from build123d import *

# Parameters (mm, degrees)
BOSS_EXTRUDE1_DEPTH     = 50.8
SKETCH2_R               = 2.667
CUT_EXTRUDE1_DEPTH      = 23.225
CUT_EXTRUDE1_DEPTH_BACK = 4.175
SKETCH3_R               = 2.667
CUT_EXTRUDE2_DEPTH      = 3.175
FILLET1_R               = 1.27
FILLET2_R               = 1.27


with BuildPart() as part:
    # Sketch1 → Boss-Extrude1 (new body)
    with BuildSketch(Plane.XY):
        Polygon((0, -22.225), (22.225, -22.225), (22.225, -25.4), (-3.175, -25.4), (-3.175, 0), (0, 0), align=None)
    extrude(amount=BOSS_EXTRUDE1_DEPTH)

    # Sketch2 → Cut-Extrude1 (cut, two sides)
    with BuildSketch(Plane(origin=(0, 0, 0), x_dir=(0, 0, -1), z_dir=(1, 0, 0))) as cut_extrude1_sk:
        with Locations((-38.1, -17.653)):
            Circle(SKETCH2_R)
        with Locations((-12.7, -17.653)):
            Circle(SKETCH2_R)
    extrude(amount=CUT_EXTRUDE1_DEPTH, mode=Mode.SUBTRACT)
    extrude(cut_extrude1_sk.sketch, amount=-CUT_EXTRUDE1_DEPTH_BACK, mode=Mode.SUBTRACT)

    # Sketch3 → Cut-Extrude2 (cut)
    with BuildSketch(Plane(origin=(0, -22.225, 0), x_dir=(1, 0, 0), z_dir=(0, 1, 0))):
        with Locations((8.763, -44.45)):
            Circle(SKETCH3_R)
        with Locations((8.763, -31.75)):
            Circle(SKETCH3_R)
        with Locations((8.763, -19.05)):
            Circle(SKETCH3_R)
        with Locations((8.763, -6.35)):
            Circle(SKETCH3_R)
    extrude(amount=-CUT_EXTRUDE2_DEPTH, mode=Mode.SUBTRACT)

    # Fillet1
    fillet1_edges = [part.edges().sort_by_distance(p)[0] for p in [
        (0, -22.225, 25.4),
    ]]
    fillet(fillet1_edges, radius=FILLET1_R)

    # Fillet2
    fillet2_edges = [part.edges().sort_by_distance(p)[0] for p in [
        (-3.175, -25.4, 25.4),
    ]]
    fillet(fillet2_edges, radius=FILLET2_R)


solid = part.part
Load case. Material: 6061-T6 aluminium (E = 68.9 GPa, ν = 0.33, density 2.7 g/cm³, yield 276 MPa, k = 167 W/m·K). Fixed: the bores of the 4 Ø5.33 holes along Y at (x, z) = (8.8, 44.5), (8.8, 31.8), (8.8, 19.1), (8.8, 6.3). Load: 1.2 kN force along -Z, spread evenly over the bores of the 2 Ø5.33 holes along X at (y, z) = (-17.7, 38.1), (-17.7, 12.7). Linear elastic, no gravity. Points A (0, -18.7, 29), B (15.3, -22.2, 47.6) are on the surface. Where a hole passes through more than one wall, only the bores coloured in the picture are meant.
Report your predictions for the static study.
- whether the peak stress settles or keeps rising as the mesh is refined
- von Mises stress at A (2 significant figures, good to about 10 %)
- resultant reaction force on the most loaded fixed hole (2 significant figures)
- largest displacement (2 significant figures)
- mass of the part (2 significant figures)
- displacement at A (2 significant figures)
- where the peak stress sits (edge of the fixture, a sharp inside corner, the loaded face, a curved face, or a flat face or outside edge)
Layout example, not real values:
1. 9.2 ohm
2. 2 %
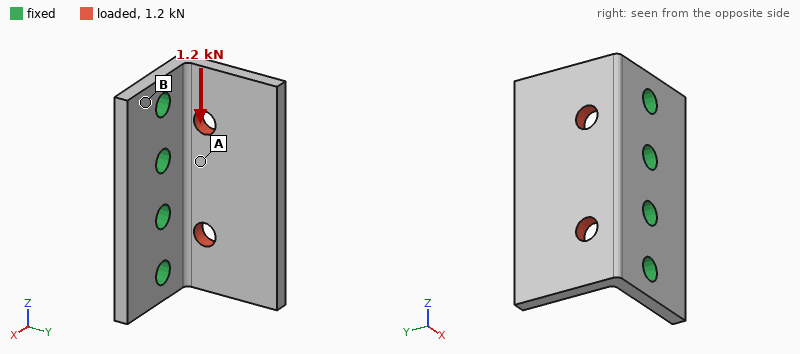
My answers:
1. keeps rising
2. 19 MPa
3. 400 N
4. 29 µm
5. 20 g
6. 6.7 µm
7. edge of the fixture
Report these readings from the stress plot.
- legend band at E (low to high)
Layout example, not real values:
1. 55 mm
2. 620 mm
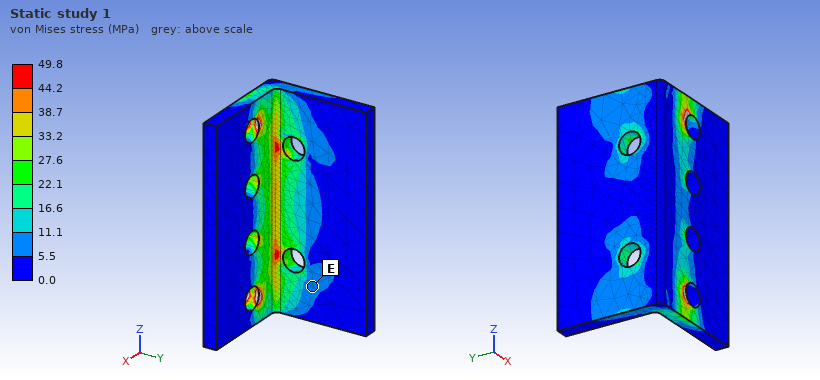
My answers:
1. 5.5 to 11.1 MPa
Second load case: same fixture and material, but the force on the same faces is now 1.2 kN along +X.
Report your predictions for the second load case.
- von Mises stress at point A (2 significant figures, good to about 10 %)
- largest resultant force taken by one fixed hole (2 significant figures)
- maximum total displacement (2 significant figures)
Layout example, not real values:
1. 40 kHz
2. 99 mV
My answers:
1. 27 MPa
2. 330 N
3. 0.18 mm
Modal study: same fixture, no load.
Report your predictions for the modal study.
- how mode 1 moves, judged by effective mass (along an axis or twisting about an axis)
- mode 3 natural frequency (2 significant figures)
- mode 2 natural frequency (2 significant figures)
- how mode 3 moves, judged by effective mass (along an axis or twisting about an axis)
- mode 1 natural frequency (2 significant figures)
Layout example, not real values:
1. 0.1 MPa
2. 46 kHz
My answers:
1. along X
2. 10 kHz
3. 5100 Hz
4. along Z
5. 3100 Hz
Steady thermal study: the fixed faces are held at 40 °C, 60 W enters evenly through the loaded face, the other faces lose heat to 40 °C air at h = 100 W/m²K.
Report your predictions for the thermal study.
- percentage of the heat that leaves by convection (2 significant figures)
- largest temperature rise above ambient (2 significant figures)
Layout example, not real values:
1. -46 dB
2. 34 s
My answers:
1. 12 %
2. 36 K
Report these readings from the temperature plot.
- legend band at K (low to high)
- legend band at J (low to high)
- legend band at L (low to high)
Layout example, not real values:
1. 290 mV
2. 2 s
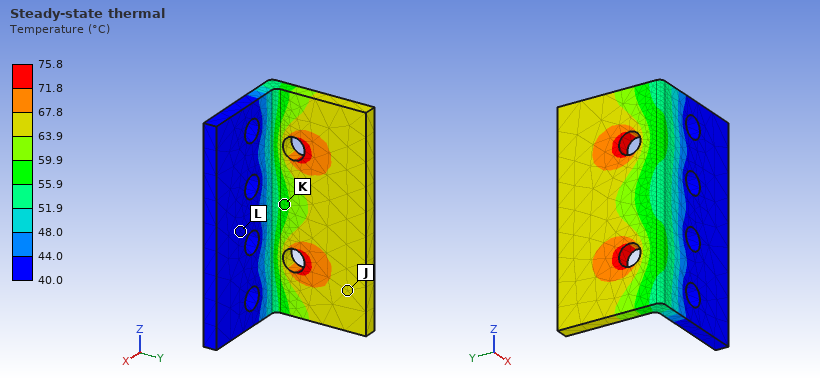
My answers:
1. 55.9 to 59.9 °C
2. 63.9 to 67.8 °C
3. 40.0 to 44.0 °C
